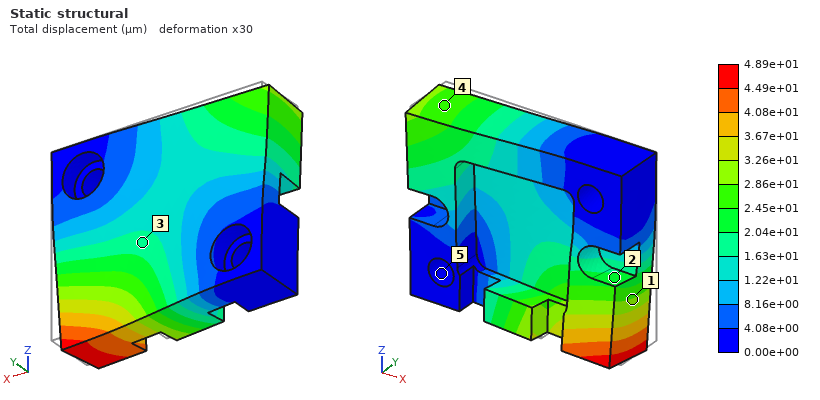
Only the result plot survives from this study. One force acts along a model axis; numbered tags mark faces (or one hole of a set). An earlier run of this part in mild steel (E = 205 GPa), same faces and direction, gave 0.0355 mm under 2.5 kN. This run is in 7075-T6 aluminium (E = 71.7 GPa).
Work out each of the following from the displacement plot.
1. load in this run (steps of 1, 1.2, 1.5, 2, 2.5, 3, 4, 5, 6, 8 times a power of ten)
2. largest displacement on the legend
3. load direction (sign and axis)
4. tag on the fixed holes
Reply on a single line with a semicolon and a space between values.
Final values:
1.2 kN; 4.89e+01 µm; -Y; 5
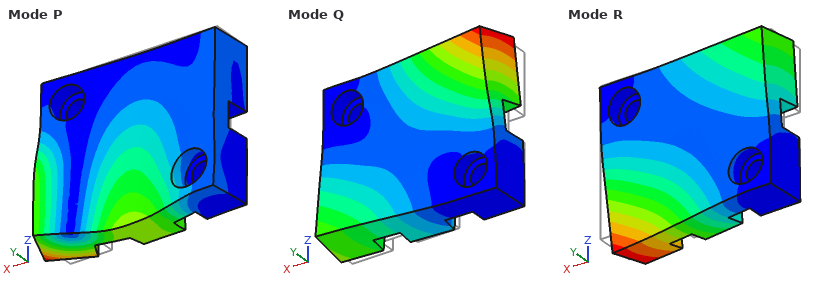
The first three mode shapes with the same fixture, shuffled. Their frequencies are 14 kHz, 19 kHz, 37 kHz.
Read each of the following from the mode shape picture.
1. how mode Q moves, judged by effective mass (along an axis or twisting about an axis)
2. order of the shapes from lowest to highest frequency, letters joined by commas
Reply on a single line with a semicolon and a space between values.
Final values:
along Y; R, Q, P
